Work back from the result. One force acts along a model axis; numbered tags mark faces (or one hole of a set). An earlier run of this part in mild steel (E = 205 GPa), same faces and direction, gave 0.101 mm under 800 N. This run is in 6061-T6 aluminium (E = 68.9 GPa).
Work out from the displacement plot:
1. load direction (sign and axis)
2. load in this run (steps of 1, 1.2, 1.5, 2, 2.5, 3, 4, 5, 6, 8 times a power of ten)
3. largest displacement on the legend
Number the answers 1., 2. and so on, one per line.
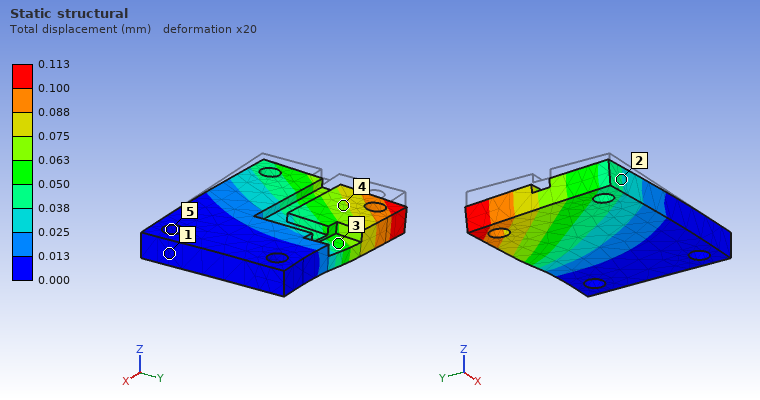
1. -Z
2. 300 N
3. 0.113 mm
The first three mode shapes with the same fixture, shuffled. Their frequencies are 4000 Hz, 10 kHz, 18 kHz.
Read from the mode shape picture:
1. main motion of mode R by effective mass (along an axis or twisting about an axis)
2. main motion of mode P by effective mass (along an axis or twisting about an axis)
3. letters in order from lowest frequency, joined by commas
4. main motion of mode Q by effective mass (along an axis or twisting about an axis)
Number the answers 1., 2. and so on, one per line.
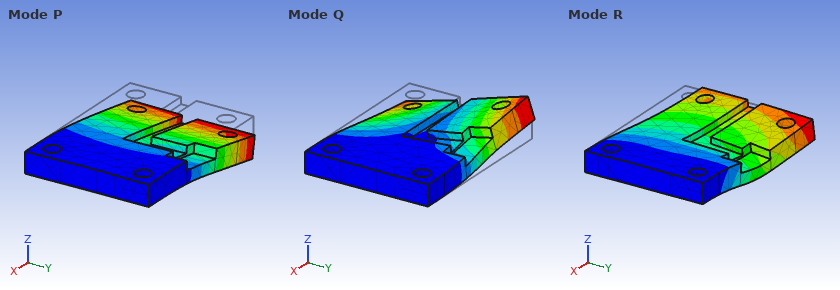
1. along Y
2. along Z
3. P, Q, R
4. twisting about X
